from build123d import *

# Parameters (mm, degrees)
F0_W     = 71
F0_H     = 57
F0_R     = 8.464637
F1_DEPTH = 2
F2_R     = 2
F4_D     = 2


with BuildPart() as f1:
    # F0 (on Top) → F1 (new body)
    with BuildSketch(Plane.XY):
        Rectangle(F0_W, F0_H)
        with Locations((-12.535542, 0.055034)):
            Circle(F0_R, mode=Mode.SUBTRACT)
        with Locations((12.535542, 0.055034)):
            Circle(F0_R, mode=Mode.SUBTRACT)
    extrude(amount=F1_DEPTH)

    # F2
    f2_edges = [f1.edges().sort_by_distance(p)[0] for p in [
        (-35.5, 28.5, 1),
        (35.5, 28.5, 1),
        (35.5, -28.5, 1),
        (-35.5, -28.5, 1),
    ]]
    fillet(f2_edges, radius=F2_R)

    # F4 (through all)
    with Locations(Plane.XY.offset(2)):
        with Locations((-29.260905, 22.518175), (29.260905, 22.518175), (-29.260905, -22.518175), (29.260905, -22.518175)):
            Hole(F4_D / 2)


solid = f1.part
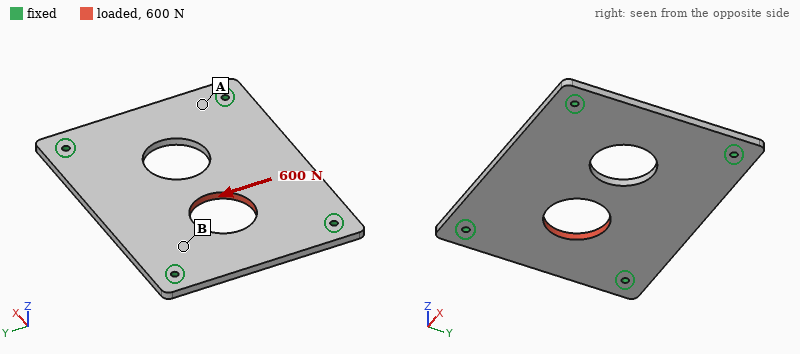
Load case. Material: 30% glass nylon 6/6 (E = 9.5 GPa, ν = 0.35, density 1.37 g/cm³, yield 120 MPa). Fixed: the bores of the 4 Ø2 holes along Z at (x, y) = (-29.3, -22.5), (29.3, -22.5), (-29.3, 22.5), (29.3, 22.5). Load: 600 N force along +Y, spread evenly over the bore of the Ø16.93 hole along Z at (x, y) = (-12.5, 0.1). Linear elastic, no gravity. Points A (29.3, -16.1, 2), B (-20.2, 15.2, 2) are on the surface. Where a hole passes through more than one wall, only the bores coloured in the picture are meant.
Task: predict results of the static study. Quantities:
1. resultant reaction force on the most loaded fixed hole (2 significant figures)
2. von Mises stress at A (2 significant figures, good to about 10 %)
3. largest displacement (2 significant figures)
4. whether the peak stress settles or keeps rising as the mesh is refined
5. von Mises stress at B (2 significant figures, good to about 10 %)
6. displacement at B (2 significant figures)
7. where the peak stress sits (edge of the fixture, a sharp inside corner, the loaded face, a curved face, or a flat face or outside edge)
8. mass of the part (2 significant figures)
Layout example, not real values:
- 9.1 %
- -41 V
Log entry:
- 230 N
- 2.8 MPa
- 35 µm
- keeps rising
- 7.6 MPa
- 19 µm
- edge of the fixture
- 9.8 g
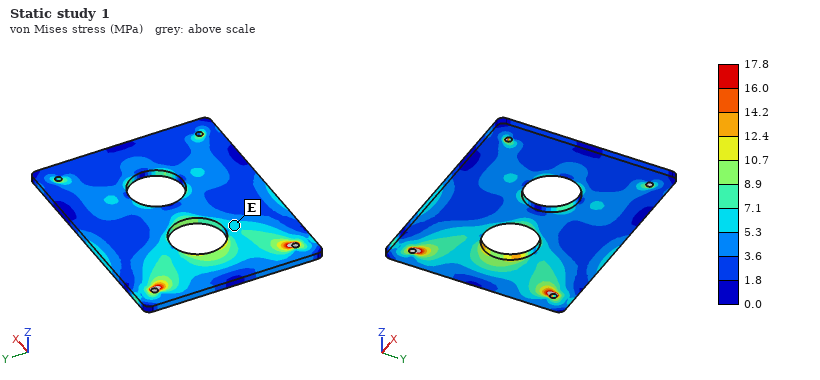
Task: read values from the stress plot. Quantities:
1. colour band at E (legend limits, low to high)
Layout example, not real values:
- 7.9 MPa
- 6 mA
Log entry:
- 5.3 to 7.1 MPa
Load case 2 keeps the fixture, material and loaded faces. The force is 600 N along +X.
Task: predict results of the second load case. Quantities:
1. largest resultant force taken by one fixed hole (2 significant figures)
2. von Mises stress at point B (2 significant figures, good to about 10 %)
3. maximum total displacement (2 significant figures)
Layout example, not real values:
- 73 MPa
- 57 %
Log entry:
- 190 N
- 5.7 MPa
- 33 µm
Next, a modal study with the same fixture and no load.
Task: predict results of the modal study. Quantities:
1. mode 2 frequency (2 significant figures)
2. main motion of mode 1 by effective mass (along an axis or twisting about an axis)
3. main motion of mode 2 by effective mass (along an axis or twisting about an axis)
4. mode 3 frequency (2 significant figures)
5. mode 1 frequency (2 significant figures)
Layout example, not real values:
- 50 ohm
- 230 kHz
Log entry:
- 1800 Hz
- along Z
- twisting about X
- 2300 Hz
- 1300 Hz
